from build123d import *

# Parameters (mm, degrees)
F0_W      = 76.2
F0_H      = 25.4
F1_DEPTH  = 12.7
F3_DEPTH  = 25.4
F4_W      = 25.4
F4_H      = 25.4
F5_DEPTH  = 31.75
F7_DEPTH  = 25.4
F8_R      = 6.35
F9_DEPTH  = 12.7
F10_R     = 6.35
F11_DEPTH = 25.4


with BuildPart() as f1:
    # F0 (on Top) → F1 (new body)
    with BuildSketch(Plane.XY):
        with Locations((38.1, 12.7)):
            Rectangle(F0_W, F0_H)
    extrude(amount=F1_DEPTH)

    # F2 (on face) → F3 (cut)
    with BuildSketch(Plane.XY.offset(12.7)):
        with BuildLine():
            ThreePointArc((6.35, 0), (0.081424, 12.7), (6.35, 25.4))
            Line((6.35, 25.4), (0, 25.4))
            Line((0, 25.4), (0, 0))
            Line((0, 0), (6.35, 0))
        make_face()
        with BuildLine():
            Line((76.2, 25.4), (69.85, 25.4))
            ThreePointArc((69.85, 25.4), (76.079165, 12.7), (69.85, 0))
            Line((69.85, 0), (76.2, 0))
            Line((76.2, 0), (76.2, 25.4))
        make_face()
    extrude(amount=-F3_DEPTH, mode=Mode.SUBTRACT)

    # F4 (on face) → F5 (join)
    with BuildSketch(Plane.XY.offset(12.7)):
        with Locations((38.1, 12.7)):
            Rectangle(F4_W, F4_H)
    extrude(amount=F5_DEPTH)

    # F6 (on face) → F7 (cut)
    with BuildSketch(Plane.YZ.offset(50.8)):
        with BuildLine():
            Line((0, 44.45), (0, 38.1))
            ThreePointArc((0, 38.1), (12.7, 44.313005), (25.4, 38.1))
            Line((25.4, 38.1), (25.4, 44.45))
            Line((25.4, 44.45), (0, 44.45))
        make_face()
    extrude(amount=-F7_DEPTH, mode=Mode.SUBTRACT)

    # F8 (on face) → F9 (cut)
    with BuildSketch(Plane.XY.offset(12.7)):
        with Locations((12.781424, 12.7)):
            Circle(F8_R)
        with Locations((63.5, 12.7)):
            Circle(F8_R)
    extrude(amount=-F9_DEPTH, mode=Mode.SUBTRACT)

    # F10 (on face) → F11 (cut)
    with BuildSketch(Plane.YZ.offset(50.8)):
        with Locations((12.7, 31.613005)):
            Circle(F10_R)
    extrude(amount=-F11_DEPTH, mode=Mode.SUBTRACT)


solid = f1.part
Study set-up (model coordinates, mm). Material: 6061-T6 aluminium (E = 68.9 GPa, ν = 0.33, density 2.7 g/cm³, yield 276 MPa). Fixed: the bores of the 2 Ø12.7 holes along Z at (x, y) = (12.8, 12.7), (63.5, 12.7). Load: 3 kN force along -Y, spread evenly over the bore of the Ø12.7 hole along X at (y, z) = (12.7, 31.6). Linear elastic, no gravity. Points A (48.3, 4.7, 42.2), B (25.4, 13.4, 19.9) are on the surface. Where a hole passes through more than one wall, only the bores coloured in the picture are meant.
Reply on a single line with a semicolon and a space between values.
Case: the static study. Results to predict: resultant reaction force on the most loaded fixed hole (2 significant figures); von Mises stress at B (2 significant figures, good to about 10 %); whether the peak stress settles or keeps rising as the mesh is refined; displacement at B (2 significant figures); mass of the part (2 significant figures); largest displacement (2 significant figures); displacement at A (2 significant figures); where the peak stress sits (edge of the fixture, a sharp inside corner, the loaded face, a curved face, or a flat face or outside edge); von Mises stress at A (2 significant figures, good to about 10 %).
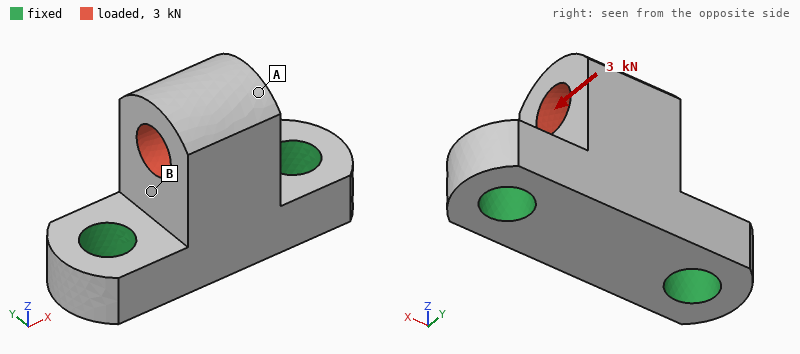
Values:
1.5 kN; 23 MPa; keeps rising; 22 µm; 97 g; 65 µm; 64 µm; edge of the fixture; 8.8 MPa
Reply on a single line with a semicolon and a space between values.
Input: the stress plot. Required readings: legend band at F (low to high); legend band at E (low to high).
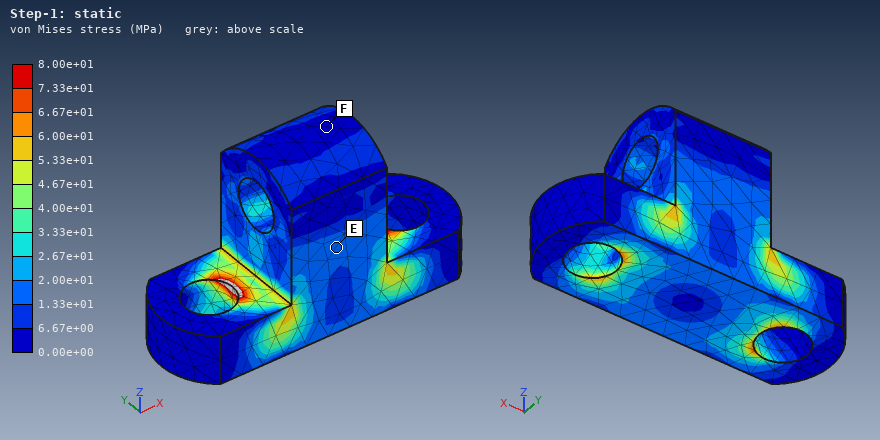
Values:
0.00e+00 to 6.67e+00 MPa; 1.33e+01 to 2.00e+01 MPa
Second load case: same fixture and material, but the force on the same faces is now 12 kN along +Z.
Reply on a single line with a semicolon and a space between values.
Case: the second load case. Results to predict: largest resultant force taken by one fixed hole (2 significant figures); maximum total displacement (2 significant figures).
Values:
6.3 kN; 27 µm
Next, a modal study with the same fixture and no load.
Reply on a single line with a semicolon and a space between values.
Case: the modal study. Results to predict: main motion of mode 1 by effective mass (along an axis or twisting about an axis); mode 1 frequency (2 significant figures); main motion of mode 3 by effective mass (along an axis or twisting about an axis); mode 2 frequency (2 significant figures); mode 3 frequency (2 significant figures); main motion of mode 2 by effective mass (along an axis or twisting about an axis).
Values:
along Y; 6700 Hz; along Z; 12 kHz; 17 kHz; along X
